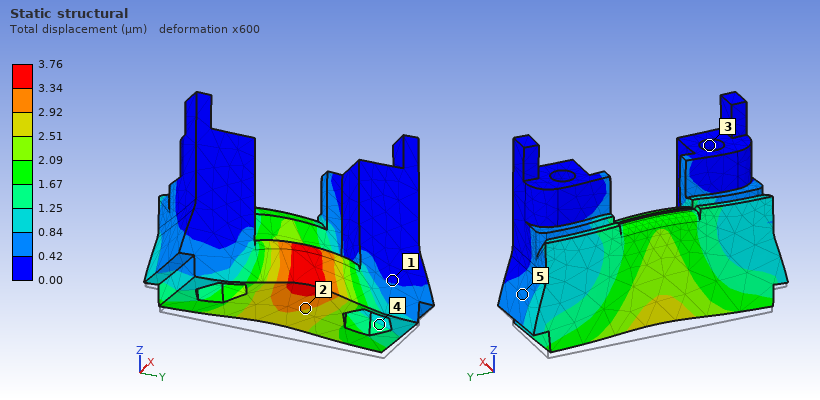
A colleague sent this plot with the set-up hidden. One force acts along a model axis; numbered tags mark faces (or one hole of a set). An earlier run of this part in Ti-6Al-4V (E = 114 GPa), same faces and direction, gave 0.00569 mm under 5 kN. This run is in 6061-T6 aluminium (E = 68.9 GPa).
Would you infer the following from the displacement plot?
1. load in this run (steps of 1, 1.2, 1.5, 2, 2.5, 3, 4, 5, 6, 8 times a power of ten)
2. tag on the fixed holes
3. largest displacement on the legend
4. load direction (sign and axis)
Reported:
2 kN
3
3.76 µm
+Z
